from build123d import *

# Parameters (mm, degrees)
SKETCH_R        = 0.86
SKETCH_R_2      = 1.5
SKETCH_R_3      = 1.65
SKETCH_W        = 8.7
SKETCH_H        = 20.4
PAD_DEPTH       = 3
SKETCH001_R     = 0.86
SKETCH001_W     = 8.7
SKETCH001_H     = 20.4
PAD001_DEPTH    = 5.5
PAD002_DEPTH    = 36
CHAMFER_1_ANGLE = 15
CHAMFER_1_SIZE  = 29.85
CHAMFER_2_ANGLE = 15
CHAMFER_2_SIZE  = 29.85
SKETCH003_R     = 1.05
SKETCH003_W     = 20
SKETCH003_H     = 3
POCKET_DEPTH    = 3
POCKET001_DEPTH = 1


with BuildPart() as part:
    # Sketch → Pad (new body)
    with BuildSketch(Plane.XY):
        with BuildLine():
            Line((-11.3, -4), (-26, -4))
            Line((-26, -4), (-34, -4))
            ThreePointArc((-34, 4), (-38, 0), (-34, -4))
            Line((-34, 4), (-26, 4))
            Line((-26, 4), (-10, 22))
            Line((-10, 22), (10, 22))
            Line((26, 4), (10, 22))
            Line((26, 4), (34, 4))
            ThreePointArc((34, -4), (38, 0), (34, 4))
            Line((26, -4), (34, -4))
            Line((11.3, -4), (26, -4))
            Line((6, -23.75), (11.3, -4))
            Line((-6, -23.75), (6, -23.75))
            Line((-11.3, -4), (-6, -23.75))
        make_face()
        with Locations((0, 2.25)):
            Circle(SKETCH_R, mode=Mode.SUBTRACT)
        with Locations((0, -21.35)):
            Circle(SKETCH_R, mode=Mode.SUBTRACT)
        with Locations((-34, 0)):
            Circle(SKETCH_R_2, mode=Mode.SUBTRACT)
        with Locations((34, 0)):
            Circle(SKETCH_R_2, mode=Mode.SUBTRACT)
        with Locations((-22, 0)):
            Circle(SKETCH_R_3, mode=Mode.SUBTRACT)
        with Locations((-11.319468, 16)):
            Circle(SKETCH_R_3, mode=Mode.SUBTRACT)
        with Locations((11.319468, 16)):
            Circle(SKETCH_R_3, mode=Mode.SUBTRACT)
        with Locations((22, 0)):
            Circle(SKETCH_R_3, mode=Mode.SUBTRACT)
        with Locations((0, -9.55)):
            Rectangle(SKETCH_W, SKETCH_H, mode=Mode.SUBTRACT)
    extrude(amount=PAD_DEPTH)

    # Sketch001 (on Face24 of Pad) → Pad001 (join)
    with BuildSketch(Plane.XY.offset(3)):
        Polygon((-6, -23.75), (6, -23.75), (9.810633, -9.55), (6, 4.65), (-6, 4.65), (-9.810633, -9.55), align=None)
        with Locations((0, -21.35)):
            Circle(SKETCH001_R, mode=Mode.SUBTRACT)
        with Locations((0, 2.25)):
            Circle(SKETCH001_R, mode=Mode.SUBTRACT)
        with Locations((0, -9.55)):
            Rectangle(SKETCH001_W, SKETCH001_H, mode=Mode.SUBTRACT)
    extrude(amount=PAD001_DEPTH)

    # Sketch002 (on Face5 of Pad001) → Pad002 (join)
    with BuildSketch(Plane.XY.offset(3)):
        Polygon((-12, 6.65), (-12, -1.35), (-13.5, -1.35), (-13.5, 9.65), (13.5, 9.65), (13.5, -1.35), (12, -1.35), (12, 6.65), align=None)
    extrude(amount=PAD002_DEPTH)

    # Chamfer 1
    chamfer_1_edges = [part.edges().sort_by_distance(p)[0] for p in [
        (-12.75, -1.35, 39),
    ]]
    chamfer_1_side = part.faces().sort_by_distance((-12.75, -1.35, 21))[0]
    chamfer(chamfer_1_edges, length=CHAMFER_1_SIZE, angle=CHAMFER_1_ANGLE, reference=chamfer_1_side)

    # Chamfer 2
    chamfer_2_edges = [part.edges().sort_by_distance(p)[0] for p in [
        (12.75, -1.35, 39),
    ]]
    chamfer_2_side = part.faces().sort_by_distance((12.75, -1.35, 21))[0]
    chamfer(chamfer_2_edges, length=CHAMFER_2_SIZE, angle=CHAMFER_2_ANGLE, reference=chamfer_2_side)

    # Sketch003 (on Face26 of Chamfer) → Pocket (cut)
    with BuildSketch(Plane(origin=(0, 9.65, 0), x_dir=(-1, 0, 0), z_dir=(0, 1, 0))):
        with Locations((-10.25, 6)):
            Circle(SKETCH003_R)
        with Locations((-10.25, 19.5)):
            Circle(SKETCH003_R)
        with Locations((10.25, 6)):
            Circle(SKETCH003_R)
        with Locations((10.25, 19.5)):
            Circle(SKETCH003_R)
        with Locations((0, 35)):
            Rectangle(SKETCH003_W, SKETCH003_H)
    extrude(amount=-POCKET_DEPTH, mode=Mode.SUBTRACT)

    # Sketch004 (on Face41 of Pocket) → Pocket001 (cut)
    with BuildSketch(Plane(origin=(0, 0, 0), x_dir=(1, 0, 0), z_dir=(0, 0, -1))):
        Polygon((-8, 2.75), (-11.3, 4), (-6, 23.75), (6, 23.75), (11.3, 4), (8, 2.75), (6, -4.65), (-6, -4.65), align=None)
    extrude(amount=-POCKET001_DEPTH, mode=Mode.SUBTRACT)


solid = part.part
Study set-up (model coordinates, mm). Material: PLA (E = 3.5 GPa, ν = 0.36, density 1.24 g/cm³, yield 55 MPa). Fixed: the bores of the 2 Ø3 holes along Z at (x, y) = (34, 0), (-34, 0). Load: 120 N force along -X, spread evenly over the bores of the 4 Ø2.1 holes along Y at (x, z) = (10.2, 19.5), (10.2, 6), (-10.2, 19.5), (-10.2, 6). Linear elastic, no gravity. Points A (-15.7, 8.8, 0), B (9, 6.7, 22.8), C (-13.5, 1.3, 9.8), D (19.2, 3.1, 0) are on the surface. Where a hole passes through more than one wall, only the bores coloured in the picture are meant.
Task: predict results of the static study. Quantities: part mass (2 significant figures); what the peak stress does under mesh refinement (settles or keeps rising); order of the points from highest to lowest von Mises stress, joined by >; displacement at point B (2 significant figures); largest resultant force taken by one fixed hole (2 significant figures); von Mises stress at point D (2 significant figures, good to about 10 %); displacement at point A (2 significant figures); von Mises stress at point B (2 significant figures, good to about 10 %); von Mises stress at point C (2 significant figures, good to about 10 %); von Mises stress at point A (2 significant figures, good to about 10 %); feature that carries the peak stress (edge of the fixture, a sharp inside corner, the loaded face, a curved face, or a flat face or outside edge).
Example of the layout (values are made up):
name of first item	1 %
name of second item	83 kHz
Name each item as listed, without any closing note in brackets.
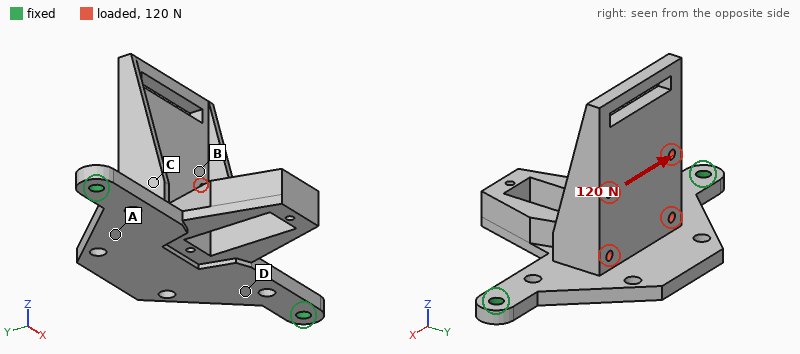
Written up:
part mass	10 g
what the peak stress does under mesh refinement	keeps rising
order of the points from highest to lowest von Mises stress, joined by >	A > D > C > B
displacement at point B	0.35 mm
largest resultant force taken by one fixed hole	68 N
von Mises stress at point D	6.1 MPa
displacement at point A	0.19 mm
von Mises stress at point B	1.4 MPa
von Mises stress at point C	2.4 MPa
von Mises stress at point A	8.9 MPa
feature that carries the peak stress	edge of the fixture
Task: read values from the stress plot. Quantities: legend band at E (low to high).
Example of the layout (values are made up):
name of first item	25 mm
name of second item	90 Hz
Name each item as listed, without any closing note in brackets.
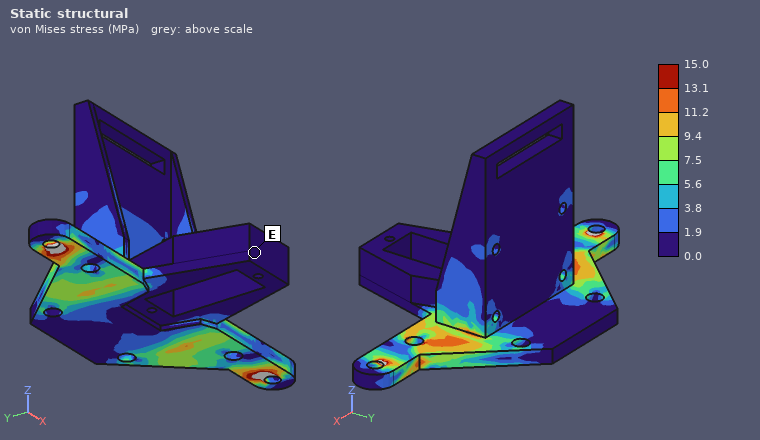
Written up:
legend band at E	0.0 to 1.9 MPa
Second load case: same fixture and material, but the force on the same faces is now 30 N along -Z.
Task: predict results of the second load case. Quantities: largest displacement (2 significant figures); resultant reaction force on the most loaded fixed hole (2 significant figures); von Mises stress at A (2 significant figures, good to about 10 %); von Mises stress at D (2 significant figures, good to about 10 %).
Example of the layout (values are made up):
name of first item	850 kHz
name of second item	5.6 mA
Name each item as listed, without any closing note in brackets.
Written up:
largest displacement	0.95 mm
resultant reaction force on the most loaded fixed hole	16 N
von Mises stress at A	5.3 MPa
von Mises stress at D	5.4 MPa
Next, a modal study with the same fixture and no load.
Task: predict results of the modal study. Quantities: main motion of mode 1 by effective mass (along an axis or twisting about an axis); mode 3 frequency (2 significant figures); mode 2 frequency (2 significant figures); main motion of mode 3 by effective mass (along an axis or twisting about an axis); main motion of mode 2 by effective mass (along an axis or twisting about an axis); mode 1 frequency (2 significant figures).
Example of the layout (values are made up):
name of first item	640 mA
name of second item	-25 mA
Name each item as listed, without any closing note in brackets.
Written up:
main motion of mode 1 by effective mass	along Y
mode 3 frequency	990 Hz
mode 2 frequency	630 Hz
main motion of mode 3 by effective mass	along X
main motion of mode 2 by effective mass	along Z
mode 1 frequency	290 Hz
